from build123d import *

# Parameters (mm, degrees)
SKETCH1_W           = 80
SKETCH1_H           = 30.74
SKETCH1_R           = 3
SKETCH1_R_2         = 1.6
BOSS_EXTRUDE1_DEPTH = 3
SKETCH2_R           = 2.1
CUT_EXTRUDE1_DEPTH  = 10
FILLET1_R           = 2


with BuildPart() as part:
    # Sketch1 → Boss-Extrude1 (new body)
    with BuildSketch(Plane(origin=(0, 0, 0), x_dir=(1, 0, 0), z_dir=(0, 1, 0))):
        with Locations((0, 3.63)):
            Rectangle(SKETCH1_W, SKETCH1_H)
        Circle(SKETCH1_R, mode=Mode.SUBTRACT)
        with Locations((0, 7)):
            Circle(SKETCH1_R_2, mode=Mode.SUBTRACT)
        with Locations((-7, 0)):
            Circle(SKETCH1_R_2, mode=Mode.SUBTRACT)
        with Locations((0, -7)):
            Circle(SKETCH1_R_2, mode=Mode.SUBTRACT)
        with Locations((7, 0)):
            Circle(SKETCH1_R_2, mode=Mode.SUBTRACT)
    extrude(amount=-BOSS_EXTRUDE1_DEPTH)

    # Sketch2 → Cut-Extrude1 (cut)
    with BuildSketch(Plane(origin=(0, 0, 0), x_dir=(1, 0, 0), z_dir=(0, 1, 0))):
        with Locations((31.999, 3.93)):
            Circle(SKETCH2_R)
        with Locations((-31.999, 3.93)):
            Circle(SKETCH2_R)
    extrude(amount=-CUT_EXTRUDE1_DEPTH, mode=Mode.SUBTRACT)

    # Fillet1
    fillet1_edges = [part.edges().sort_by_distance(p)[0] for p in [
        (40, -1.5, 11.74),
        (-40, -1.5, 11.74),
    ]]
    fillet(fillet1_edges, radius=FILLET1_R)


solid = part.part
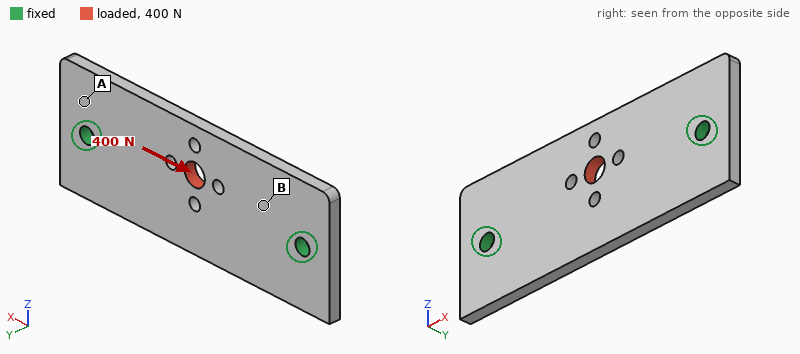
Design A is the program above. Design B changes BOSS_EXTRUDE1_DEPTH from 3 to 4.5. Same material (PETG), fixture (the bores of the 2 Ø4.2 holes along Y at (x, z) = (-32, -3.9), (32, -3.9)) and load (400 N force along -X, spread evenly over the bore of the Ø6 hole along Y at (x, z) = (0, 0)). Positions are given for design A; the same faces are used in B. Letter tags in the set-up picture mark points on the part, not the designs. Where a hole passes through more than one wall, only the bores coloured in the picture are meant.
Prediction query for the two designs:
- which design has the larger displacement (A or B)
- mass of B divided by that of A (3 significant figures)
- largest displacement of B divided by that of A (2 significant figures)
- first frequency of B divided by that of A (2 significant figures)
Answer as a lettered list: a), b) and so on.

a) A
b) 1.50
c) 0.67
d) 1.4
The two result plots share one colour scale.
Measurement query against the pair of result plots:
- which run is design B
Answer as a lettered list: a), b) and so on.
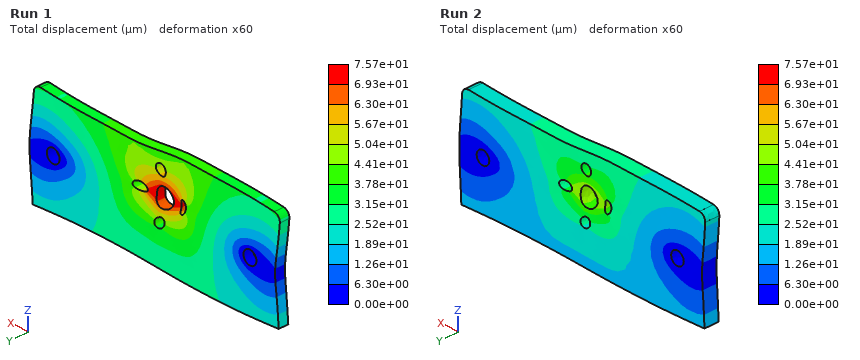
a) Run 2
